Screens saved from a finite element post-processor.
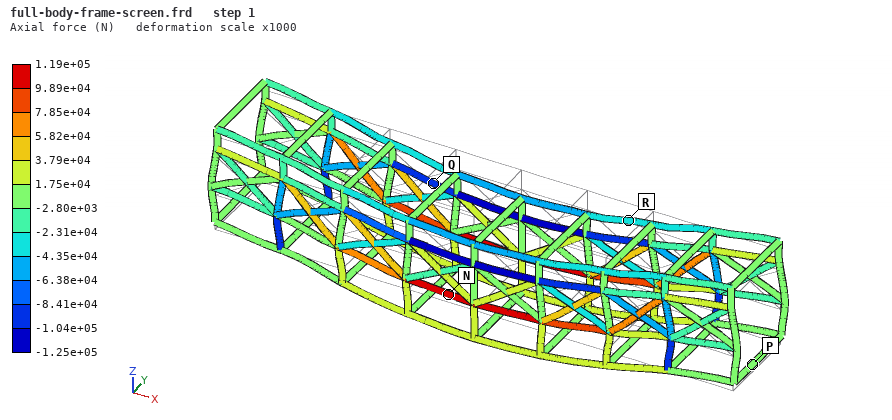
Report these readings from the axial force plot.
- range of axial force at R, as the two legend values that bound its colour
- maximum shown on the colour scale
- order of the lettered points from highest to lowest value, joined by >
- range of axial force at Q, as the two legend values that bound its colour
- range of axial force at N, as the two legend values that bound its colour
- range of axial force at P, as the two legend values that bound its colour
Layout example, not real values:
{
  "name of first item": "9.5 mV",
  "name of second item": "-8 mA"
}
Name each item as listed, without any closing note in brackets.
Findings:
{
  "range of axial force at R, as the two legend values that bound its colour": "-4.35e+04 to -2.31e+04 N",
  "maximum shown on the colour scale": "1.19e+05 N",
  "order of the lettered points from highest to lowest value, joined by >": "N > P > R > Q",
  "range of axial force at Q, as the two legend values that bound its colour": "-1.04e+05 to -8.41e+04 N",
  "range of axial force at N, as the two legend values that bound its colour": "9.89e+04 to 1.19e+05 N",
  "range of axial force at P, as the two legend values that bound its colour": "-2.80e+03 to 1.75e+04 N"
}
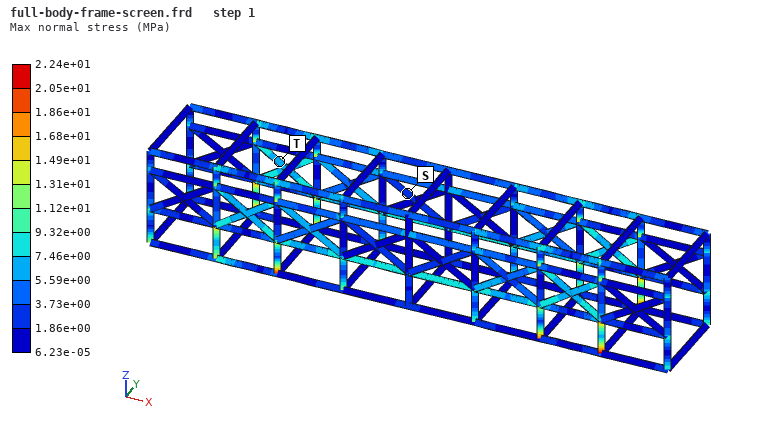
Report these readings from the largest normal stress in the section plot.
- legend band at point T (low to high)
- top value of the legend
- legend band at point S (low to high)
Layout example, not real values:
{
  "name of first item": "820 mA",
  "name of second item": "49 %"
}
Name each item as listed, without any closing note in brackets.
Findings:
{
  "legend band at point T": "5.59e+00 to 7.46e+00 MPa",
  "top value of the legend": "2.24e+01 MPa",
  "legend band at point S": "1.86e+00 to 3.73e+00 MPa"
}
